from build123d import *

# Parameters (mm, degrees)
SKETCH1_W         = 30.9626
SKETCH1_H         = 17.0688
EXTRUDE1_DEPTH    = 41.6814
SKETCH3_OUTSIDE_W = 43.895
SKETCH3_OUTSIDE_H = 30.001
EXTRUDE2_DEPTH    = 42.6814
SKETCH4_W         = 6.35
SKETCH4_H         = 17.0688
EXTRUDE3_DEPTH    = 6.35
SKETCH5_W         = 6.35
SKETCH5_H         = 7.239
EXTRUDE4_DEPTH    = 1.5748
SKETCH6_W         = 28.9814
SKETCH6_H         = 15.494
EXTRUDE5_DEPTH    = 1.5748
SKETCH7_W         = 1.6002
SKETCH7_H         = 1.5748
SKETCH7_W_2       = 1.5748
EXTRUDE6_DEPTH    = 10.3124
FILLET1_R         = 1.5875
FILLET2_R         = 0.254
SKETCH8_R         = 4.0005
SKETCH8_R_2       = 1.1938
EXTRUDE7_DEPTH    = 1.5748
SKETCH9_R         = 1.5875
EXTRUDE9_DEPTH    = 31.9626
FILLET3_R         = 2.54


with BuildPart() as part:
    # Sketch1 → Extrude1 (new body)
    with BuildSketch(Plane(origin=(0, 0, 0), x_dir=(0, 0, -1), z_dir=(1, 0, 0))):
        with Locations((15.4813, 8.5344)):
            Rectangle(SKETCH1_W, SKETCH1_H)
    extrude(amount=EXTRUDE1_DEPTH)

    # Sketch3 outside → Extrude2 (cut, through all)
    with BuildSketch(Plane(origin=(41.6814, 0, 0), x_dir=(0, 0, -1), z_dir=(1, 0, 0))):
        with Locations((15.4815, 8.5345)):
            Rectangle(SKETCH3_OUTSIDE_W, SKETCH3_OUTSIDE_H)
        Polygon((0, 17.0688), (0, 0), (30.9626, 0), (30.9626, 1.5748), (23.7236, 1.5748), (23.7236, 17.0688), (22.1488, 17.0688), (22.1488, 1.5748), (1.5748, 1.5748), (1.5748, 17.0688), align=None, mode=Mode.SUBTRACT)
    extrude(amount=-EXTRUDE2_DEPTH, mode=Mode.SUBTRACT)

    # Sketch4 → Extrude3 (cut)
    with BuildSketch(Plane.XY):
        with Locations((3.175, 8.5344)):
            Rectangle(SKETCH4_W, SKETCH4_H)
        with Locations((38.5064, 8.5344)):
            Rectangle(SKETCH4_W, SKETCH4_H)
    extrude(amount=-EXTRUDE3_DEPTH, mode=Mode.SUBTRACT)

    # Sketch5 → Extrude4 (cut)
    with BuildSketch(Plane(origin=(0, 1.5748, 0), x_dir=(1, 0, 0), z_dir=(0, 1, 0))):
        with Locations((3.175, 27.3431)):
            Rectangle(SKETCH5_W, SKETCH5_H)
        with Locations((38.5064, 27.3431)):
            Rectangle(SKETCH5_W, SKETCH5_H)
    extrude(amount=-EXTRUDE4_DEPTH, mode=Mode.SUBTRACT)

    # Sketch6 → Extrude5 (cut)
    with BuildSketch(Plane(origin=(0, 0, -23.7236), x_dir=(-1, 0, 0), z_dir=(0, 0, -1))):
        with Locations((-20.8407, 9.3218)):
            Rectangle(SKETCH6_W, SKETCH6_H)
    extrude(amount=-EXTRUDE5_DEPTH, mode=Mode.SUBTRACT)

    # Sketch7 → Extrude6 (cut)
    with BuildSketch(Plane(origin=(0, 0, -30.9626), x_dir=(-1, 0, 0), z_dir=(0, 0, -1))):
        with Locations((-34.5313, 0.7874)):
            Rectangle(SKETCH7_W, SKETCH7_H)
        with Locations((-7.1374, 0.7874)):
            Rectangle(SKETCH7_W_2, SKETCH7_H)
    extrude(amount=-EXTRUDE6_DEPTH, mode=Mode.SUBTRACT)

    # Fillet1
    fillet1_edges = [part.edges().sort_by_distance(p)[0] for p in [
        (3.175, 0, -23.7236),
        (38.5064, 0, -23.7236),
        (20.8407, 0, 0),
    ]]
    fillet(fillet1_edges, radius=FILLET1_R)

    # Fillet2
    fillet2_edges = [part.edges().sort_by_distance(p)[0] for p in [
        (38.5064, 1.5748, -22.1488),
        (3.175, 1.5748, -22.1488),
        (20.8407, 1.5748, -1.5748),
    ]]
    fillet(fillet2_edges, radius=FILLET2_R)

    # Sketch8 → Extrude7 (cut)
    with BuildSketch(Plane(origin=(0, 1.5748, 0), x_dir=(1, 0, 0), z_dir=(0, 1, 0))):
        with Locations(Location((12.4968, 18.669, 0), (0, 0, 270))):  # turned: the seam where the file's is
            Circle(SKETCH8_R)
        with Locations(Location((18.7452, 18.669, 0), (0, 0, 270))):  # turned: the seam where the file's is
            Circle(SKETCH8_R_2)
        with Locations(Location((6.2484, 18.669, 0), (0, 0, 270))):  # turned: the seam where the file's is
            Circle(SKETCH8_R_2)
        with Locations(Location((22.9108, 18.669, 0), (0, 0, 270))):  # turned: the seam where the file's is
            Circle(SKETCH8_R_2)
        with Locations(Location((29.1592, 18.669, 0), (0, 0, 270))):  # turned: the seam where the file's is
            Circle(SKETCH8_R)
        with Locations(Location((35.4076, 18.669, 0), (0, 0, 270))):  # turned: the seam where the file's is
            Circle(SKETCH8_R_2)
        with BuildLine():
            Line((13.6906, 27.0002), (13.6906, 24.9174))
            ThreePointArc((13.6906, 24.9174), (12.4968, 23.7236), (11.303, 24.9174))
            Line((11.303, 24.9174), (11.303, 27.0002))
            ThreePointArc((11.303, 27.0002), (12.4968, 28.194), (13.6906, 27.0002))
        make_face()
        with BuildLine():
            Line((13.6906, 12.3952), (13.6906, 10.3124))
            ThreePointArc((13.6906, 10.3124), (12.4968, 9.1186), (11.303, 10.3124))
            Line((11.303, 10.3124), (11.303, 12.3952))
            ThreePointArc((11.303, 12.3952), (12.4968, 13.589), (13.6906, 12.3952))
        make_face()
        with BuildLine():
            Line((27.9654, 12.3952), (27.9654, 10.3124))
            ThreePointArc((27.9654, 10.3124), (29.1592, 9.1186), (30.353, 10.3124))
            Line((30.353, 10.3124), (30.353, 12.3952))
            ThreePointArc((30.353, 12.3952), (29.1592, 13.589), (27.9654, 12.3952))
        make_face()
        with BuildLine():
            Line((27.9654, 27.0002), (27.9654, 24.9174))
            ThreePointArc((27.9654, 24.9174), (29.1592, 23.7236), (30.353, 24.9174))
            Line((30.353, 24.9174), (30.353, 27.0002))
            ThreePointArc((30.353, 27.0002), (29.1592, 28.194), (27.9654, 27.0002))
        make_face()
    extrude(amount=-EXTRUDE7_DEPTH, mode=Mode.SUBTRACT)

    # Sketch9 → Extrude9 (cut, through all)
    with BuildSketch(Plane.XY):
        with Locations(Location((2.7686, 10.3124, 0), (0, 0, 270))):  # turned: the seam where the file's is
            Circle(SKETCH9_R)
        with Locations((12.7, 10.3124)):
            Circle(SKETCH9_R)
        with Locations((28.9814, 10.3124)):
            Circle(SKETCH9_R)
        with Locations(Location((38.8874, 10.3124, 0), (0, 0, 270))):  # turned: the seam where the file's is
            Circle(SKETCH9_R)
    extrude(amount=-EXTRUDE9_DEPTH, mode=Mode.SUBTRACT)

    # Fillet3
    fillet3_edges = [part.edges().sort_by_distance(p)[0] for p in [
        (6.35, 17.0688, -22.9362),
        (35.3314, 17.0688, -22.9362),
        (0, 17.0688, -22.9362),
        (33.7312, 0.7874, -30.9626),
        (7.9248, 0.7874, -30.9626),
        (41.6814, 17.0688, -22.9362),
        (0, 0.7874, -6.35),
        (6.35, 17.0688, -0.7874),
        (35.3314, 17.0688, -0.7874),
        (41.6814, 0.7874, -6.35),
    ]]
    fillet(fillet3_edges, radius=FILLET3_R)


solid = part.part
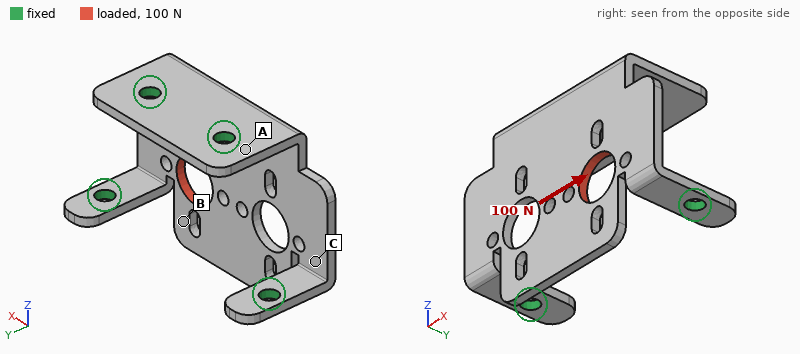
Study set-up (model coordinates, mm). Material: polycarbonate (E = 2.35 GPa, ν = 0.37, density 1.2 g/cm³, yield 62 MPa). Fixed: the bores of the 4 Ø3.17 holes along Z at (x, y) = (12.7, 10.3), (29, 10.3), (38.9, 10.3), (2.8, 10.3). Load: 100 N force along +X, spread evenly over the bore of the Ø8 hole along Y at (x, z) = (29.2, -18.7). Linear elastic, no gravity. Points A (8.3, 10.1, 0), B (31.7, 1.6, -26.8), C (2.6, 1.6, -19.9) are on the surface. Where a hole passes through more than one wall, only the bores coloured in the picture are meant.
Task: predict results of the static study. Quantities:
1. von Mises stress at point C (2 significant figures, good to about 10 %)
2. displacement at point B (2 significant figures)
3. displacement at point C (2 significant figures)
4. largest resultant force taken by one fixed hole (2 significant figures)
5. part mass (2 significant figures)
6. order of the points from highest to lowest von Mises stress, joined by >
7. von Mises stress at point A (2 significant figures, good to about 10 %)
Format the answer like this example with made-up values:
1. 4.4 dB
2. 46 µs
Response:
1. 9.6 MPa
2. 0.34 mm
3. 0.20 mm
4. 35 N
5. 2.9 g
6. C > A > B
7. 5.9 MPa
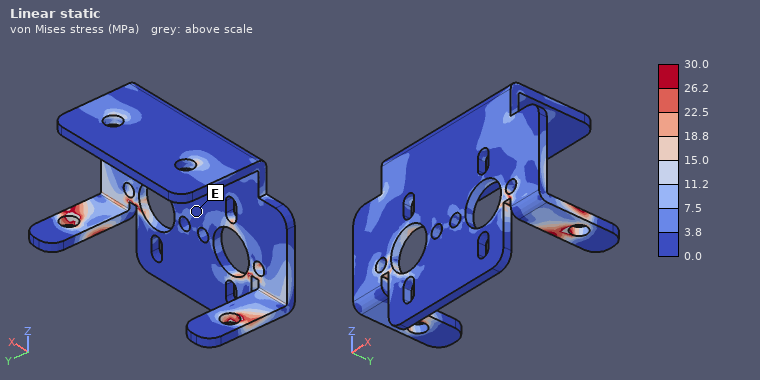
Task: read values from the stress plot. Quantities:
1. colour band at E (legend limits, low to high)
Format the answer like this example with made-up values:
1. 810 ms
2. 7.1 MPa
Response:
1. 0.0 to 3.8 MPa
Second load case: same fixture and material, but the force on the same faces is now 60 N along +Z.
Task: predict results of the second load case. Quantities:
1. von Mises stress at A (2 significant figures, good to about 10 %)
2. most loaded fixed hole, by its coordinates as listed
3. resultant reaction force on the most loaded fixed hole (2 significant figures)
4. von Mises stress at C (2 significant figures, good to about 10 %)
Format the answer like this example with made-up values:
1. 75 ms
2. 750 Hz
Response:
1. 5.1 MPa
2. (29, 10.3)
3. 24 N
4. 8.1 MPa
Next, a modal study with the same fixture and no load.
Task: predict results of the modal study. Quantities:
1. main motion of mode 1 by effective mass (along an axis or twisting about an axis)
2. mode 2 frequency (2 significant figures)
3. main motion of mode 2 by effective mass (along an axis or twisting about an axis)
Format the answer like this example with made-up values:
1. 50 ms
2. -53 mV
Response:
1. along Y
2. 1900 Hz
3. along Z
